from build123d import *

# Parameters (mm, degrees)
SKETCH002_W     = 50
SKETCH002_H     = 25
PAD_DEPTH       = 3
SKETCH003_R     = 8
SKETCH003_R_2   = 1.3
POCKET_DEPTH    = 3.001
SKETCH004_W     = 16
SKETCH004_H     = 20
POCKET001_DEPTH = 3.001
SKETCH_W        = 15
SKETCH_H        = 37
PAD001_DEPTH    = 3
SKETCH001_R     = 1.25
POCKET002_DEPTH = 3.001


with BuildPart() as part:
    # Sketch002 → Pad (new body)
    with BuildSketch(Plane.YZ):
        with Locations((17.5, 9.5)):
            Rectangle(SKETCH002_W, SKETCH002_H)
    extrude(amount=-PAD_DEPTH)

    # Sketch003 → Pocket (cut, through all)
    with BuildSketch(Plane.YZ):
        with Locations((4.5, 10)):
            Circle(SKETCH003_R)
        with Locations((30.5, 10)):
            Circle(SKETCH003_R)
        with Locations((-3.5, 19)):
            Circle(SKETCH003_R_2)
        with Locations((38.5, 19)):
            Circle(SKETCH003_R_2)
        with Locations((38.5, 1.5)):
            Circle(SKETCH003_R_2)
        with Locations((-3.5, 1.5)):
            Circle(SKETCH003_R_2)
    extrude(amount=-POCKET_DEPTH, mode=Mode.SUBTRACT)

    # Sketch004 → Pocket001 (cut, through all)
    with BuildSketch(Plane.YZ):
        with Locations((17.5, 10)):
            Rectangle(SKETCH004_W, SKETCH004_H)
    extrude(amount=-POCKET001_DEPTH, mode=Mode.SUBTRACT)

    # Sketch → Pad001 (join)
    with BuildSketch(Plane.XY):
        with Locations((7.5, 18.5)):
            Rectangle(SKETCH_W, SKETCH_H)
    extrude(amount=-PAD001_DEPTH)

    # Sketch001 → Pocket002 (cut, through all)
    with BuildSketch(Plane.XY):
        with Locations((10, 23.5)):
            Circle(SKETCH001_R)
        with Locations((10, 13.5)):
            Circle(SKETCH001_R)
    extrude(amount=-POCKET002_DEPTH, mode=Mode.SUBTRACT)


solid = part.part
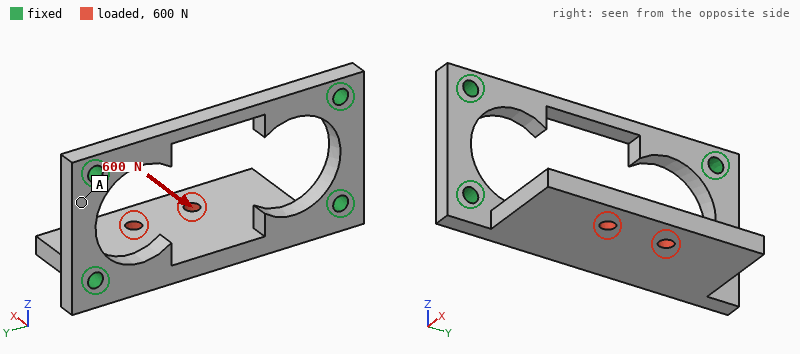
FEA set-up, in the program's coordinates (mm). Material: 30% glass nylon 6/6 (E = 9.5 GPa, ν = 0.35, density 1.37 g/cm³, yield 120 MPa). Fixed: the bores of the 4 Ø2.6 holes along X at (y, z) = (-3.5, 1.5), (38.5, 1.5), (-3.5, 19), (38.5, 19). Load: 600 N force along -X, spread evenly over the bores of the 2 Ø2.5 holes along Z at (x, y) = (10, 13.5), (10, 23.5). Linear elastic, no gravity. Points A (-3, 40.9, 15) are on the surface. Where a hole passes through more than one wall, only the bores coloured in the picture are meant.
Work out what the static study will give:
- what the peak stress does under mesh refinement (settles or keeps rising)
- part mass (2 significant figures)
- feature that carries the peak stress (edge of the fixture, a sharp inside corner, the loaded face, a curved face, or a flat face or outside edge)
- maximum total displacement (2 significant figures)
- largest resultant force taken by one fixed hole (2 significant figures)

keeps rising
4.5 g
edge of the fixture
0.29 mm
370 N
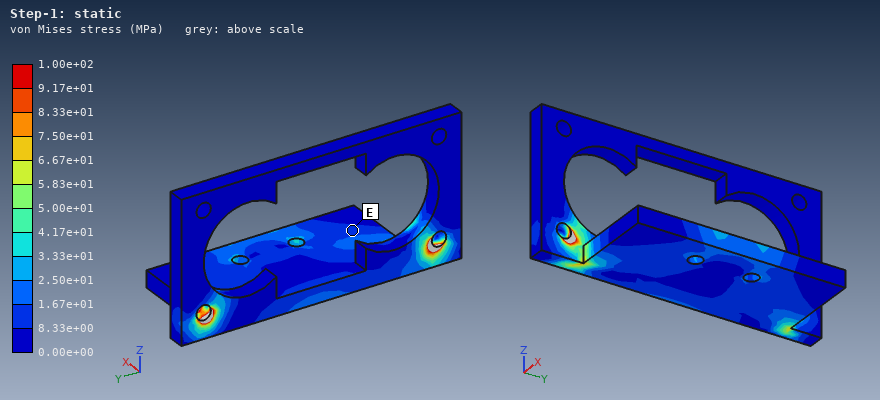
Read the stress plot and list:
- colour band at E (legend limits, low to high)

8.33e+00 to 1.67e+01 MPa
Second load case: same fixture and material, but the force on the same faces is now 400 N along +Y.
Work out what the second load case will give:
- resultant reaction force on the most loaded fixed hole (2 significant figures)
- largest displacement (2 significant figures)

240 N
70 µm
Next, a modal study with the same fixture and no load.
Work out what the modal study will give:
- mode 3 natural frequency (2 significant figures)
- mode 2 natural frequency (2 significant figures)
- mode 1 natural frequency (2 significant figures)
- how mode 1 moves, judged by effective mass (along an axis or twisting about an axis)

5800 Hz
5000 Hz
2100 Hz
along Z
